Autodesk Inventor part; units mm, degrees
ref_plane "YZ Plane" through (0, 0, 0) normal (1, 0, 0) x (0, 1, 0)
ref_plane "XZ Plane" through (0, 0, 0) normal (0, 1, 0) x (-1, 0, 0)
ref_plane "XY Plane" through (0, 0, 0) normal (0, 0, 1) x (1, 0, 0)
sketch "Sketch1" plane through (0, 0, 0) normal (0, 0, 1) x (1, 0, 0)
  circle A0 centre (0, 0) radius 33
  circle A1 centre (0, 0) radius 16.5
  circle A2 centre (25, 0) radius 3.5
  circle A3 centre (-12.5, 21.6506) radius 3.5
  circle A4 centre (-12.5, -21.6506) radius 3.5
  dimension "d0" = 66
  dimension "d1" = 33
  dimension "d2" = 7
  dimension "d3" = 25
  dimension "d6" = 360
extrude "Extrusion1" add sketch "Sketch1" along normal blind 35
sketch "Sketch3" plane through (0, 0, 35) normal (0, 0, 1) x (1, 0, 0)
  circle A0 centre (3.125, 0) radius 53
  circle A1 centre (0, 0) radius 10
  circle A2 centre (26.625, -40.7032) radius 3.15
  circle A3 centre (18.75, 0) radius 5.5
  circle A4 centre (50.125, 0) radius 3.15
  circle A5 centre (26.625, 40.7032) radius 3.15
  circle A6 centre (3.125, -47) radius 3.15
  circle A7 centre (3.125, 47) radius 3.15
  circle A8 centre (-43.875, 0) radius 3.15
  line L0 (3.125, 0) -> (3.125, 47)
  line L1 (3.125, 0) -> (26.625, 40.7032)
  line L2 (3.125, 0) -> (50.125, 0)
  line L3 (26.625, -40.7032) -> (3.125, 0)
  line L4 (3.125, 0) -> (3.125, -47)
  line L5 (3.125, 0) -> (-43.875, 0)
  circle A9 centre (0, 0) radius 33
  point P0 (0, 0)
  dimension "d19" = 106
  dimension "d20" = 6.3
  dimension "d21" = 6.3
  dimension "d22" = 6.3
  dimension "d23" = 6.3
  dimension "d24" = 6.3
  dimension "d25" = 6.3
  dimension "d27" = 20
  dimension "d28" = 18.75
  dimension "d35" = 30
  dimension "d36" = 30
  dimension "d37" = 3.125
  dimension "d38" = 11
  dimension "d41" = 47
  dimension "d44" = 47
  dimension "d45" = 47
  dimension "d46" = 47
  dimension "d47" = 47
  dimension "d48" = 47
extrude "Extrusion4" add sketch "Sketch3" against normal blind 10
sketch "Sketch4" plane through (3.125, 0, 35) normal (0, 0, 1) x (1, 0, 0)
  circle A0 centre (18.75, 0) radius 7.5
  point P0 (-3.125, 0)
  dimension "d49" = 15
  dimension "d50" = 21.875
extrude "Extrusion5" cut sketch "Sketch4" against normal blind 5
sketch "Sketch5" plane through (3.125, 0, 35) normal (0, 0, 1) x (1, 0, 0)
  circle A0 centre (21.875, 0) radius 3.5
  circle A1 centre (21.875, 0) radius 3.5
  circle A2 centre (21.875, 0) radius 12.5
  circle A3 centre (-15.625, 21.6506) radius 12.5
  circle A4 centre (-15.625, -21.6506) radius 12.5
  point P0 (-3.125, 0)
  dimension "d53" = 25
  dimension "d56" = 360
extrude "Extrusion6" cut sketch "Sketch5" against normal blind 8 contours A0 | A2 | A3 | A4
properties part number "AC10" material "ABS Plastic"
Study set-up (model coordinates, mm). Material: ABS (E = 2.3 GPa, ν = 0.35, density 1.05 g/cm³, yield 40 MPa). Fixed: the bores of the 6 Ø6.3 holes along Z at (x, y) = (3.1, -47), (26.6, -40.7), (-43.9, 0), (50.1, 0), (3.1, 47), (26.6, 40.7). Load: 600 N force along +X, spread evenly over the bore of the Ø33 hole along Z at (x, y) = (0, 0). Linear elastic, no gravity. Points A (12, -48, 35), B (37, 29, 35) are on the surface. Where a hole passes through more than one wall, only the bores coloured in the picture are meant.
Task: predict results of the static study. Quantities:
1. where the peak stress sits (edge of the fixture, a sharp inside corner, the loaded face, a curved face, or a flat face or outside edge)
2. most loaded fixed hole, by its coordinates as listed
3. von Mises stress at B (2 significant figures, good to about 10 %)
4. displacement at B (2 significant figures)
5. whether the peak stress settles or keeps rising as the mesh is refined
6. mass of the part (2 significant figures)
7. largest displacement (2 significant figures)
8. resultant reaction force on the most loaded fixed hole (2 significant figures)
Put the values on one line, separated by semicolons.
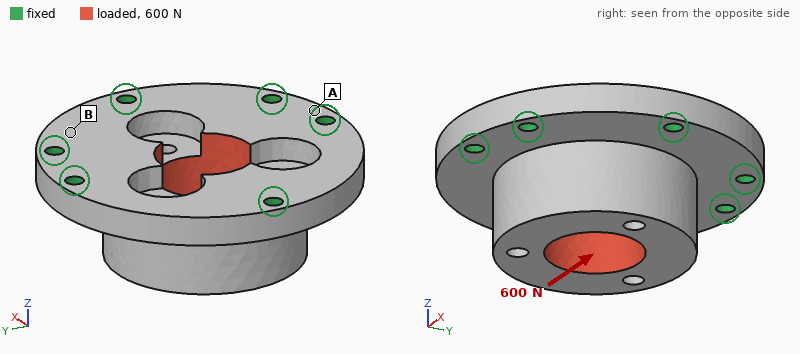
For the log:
edge of the fixture; (-43.9, 0); 0.38 MPa; 7.3 µm; keeps rising; 130 g; 28 µm; 210 N
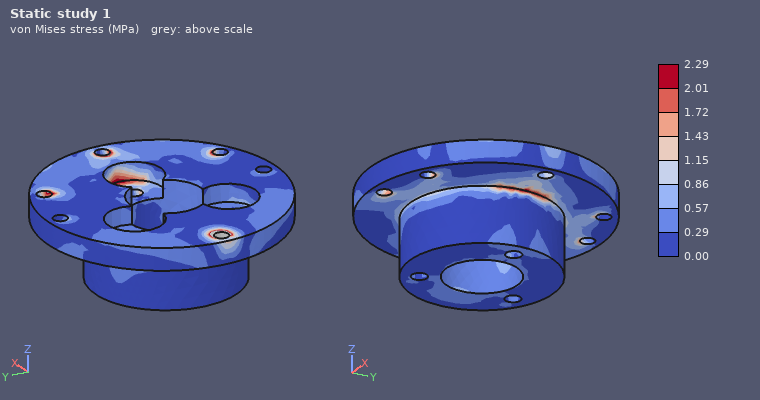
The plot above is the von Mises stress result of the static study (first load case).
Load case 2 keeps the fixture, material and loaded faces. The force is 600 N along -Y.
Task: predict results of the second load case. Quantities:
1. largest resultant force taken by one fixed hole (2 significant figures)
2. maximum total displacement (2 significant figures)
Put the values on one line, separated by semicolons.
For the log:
150 N; 26 µm
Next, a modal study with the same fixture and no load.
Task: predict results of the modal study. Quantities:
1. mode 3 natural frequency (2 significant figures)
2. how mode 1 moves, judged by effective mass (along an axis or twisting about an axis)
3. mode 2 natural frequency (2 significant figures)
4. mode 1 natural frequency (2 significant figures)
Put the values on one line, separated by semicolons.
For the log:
2700 Hz; along Z; 2600 Hz; 2400 Hz
